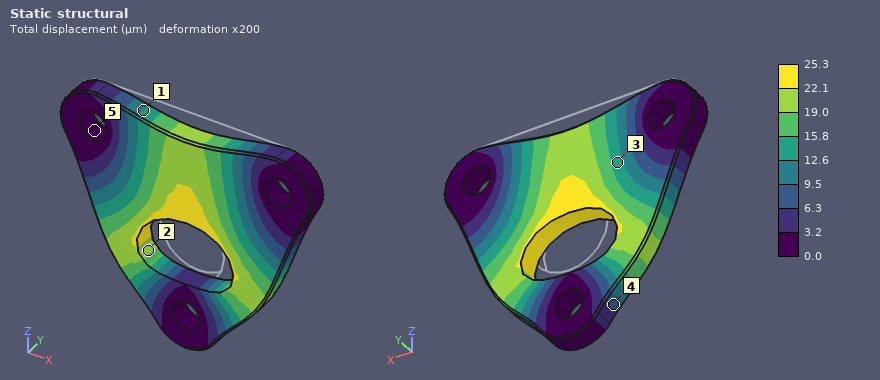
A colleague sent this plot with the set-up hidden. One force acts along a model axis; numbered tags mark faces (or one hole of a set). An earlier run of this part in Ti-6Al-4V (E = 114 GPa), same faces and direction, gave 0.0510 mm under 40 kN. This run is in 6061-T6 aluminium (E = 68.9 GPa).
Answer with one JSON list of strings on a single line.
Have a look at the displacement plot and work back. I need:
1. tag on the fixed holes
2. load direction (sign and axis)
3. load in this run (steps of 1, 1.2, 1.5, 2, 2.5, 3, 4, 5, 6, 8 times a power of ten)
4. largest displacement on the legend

["5", "-Z", "12 kN", "25.3 µm"]
